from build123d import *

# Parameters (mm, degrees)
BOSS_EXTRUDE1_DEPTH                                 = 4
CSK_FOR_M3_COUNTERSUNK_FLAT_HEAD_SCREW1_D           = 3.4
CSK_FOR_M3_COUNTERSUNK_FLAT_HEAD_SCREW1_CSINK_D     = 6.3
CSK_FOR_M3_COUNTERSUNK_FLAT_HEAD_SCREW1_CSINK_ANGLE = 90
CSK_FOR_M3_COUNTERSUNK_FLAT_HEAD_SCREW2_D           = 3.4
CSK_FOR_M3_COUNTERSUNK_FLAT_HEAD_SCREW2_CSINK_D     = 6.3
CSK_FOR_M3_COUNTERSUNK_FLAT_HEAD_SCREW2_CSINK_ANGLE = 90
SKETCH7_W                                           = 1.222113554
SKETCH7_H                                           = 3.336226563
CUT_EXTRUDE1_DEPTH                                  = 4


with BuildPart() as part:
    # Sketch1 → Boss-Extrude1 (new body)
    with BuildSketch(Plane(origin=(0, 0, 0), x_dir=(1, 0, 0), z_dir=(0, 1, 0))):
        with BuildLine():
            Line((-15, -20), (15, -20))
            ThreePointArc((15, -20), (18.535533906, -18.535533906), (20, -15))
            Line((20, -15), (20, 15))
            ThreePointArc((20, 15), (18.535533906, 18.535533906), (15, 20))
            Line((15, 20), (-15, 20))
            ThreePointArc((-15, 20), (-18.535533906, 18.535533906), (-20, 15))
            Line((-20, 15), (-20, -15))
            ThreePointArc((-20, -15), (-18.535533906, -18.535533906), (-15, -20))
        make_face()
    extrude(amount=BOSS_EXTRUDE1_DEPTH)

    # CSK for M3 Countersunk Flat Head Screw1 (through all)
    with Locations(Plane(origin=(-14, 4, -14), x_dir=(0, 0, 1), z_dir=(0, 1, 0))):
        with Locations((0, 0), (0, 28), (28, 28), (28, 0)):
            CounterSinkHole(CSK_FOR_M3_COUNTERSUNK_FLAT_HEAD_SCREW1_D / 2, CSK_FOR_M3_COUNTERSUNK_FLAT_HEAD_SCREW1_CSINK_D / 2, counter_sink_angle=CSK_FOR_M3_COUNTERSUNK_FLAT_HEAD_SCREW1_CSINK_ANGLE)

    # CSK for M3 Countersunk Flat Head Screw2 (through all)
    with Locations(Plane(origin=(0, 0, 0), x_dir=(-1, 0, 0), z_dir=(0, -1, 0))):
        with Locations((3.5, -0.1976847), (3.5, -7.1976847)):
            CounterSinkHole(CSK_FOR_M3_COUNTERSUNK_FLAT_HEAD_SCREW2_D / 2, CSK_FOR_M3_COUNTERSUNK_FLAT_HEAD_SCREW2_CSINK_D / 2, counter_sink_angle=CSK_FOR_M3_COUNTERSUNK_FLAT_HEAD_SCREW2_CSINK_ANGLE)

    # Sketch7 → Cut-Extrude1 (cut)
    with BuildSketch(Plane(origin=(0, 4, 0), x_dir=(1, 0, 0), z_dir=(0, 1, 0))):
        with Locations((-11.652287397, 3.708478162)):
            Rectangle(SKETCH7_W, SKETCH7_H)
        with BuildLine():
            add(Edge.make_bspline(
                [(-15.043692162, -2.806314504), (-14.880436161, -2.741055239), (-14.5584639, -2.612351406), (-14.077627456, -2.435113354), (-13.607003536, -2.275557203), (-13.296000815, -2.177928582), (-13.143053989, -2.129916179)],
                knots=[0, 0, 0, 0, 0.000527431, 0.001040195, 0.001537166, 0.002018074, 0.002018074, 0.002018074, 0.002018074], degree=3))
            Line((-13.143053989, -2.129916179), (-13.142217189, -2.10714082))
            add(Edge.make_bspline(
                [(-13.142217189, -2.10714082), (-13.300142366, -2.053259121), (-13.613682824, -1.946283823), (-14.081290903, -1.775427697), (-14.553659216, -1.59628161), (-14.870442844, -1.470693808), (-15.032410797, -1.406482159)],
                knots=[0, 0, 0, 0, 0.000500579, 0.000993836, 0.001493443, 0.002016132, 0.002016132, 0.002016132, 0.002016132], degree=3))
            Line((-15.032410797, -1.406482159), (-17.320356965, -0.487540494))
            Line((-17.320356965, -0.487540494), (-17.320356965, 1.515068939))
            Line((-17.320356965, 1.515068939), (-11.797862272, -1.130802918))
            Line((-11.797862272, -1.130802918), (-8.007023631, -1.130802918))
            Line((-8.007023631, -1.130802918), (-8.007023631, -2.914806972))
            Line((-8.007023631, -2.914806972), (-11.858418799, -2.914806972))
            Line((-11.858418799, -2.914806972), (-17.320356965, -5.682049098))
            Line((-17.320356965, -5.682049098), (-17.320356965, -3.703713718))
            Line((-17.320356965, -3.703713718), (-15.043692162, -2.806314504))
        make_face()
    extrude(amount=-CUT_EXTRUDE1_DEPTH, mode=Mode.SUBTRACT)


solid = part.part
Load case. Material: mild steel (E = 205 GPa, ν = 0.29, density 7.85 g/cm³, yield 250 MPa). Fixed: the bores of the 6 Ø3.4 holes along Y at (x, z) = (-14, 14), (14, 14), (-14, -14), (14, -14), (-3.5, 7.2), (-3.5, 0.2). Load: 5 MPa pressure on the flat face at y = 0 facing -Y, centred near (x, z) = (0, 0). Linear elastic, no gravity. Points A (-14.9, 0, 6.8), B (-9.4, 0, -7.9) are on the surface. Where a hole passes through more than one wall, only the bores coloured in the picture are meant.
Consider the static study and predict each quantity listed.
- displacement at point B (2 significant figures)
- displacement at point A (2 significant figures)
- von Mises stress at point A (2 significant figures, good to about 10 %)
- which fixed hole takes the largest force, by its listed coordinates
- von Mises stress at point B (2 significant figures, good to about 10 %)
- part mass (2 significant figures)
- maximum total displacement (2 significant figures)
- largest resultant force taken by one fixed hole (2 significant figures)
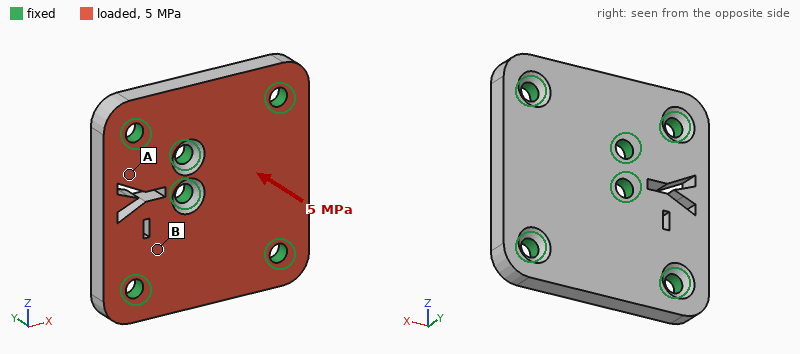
3.3 µm
3.5 µm
26 MPa
(14, -14)
59 MPa
46 g
11 µm
1.6 kN
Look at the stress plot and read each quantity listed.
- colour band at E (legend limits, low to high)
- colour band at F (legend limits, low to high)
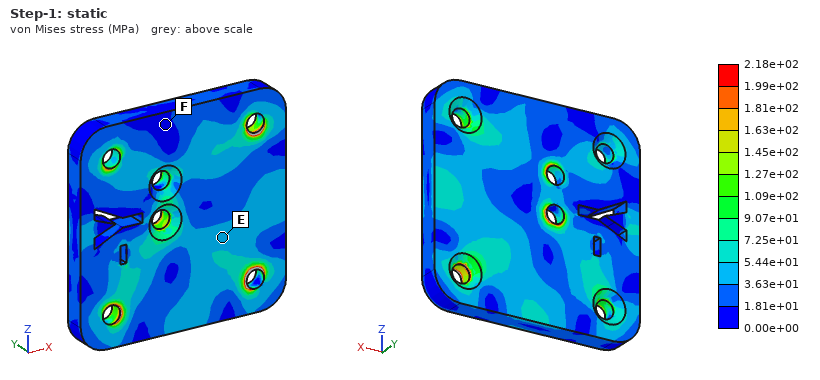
3.63e+01 to 5.44e+01 MPa
0.00e+00 to 1.81e+01 MPa
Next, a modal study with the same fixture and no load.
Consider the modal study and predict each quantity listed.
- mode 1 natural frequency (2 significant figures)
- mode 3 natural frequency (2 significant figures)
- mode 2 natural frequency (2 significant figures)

23 kHz
26 kHz
23 kHz
